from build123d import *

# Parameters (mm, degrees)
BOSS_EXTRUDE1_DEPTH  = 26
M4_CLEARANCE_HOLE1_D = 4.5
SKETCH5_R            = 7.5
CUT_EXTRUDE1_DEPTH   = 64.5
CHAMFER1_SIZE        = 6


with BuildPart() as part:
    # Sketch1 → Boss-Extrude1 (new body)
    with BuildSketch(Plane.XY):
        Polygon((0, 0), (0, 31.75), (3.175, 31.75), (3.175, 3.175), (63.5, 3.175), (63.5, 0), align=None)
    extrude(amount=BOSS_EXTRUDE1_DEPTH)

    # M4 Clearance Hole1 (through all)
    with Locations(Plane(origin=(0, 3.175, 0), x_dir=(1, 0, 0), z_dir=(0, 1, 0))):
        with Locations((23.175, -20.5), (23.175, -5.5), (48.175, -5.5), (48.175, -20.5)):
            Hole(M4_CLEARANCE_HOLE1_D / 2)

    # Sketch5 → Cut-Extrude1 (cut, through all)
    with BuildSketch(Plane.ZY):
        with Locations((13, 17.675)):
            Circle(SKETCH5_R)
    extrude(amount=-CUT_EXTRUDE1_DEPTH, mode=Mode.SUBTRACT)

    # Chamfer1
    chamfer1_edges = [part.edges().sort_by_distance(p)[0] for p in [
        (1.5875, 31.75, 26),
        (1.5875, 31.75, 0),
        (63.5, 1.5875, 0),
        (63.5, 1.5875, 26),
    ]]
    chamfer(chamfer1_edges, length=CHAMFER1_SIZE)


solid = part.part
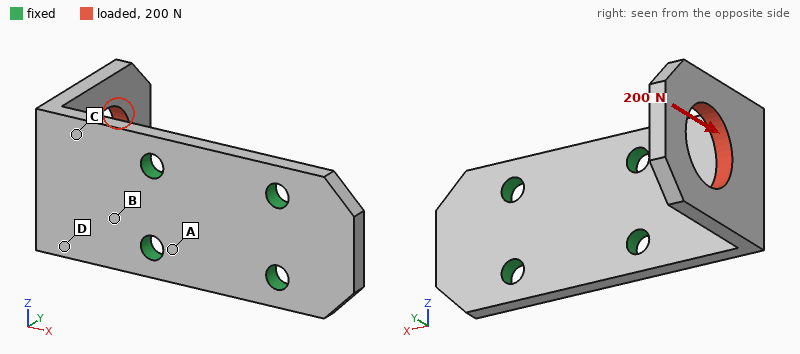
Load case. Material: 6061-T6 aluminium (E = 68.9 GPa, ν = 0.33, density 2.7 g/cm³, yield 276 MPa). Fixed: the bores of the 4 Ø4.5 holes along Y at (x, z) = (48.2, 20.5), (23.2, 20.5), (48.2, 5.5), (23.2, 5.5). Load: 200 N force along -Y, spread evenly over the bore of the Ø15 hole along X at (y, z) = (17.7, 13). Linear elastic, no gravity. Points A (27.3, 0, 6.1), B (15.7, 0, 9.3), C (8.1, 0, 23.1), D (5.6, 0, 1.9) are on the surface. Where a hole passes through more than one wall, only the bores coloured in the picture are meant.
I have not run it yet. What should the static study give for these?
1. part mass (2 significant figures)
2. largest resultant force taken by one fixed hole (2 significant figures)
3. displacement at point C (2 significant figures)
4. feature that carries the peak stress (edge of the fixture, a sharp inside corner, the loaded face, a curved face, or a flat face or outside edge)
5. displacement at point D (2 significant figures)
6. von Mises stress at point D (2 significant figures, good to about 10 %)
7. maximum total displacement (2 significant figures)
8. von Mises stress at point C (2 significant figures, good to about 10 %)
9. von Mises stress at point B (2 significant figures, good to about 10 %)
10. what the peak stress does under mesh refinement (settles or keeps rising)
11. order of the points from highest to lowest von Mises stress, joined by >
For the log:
18 g
100 N
0.063 mm
edge of the fixture
0.083 mm
19 MPa
0.28 mm
30 MPa
57 MPa
keeps rising
B > C > D > A
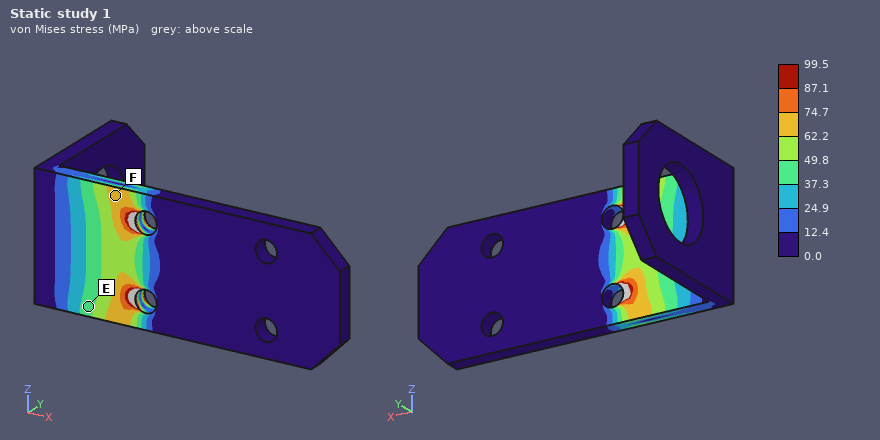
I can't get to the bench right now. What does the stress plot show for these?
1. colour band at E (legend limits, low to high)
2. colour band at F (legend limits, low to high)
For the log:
37.3 to 49.8 MPa
62.2 to 74.7 MPa
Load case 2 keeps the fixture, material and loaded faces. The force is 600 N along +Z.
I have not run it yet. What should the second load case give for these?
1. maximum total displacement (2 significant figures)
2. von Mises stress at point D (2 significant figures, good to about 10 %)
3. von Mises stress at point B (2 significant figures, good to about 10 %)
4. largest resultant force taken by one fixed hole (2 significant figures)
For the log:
0.55 mm
120 MPa
110 MPa
900 N
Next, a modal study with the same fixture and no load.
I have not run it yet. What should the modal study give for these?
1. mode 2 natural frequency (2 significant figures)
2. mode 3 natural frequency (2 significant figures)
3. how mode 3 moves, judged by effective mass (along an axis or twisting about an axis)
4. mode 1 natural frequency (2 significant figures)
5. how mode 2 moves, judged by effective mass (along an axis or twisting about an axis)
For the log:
2800 Hz
4200 Hz
along Y
1600 Hz
along Z
